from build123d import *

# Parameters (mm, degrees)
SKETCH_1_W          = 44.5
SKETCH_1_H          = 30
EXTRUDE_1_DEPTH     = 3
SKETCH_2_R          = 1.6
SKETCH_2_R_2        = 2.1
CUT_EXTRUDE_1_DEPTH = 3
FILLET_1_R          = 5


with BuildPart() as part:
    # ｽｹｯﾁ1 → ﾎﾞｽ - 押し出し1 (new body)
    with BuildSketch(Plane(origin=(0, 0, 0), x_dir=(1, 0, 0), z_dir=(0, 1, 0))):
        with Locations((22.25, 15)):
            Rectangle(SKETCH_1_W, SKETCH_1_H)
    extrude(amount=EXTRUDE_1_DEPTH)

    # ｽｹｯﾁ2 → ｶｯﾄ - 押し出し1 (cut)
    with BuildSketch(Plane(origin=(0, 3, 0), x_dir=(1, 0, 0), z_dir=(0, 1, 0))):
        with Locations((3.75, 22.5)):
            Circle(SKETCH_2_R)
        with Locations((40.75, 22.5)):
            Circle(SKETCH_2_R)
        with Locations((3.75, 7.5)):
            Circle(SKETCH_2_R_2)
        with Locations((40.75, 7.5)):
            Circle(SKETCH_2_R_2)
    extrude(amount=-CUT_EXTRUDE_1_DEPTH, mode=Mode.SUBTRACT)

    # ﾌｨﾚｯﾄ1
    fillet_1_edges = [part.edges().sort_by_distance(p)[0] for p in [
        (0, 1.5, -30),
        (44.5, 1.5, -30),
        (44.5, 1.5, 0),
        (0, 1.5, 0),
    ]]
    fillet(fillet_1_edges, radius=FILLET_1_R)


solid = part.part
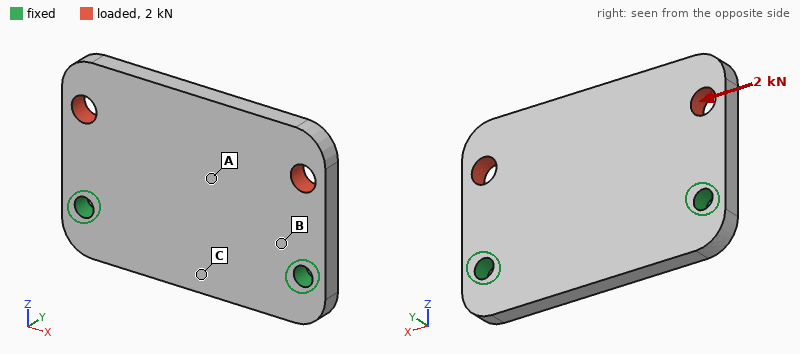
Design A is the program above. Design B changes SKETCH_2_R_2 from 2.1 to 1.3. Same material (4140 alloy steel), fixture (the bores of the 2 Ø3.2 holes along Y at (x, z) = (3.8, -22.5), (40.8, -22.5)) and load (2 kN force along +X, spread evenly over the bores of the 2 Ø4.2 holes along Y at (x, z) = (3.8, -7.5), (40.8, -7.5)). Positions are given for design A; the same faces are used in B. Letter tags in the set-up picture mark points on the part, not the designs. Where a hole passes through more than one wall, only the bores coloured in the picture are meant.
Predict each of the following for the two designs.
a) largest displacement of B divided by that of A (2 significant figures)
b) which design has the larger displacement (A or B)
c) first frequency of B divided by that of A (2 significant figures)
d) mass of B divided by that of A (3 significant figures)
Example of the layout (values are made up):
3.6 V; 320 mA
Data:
0.91; A; 1.00; 1.01
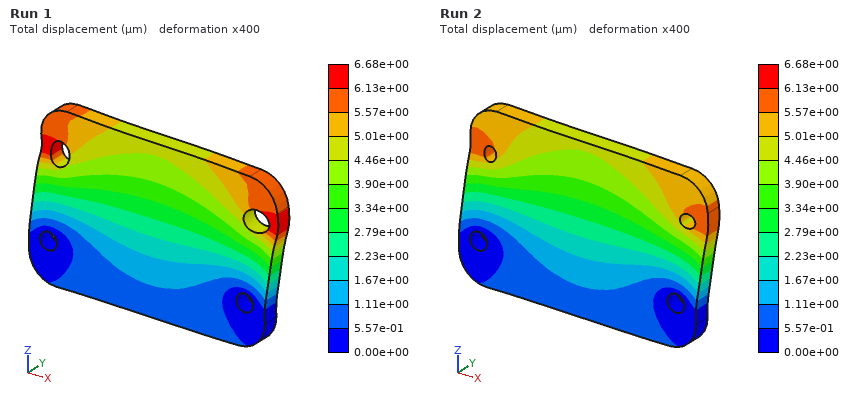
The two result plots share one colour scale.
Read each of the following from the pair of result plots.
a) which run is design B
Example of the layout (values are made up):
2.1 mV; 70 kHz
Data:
Run 2
